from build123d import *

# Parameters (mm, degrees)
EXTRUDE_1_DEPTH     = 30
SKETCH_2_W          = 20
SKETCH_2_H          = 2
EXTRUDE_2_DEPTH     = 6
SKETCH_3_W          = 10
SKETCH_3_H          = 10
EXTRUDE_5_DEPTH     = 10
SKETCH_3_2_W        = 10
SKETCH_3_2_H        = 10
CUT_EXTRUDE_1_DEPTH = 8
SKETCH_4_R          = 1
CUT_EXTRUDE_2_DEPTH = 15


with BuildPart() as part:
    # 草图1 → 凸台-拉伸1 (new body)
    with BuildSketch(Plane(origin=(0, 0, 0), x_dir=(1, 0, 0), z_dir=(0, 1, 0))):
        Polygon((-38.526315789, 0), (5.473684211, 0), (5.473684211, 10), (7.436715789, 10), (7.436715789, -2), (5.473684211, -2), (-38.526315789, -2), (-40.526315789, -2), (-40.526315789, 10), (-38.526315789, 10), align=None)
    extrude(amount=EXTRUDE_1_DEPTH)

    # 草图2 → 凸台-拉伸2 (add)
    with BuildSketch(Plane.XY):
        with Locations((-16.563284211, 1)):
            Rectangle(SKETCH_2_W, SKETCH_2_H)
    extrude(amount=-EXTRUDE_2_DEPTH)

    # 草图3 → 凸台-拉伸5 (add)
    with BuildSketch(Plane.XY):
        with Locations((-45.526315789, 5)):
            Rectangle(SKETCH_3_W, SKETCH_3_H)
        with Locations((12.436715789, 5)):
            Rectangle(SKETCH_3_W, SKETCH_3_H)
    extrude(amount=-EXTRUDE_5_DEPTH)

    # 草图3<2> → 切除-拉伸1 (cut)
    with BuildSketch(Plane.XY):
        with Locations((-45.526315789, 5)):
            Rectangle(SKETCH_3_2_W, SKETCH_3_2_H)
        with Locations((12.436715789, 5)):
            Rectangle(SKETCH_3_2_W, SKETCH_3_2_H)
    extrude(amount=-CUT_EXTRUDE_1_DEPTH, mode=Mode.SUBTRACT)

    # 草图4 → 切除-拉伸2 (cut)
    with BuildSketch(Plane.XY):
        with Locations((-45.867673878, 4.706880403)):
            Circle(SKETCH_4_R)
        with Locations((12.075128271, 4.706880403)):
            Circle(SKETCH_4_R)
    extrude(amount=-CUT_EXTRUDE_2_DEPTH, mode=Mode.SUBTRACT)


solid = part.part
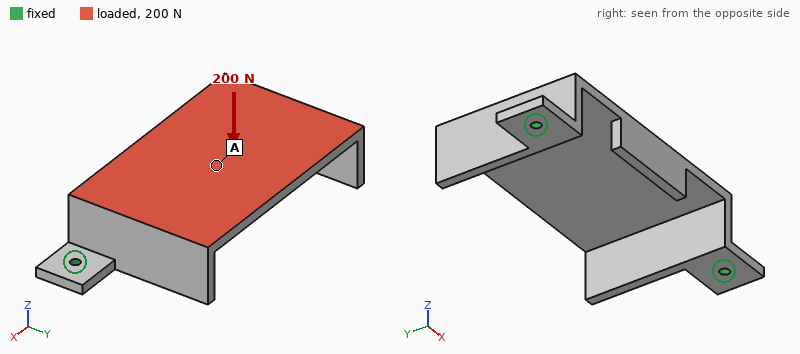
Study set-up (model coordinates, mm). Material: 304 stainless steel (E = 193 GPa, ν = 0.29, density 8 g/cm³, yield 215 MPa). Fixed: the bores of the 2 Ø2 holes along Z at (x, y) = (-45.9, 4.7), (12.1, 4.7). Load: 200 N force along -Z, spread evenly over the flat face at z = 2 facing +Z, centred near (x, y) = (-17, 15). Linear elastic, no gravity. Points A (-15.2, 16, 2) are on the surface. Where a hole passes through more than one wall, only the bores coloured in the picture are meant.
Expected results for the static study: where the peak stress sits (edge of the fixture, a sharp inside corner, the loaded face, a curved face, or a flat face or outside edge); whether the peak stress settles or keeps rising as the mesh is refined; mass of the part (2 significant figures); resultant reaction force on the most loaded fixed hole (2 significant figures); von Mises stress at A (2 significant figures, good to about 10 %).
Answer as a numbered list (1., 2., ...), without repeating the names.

1. edge of the fixture
2. keeps rising
3. 38 g
4. 130 N
5. 19 MPa
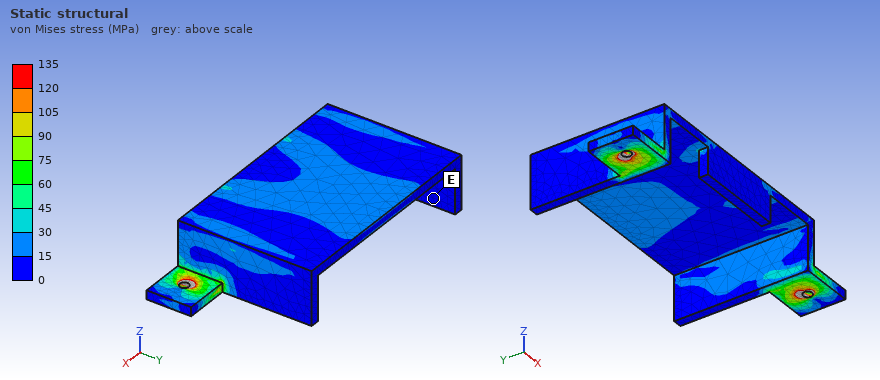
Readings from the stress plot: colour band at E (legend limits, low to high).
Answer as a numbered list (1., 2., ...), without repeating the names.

1. 0 to 15 MPa
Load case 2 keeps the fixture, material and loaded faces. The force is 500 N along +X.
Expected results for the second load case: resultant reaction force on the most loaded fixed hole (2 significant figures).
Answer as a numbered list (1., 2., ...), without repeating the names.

1. 280 N
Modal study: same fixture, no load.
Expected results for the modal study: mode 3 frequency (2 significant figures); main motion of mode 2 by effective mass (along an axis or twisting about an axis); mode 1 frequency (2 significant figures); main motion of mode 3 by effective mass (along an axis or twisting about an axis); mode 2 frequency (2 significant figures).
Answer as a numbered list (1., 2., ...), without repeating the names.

1. 3500 Hz
2. along X
3. 1500 Hz
4. along X
5. 2600 Hz
